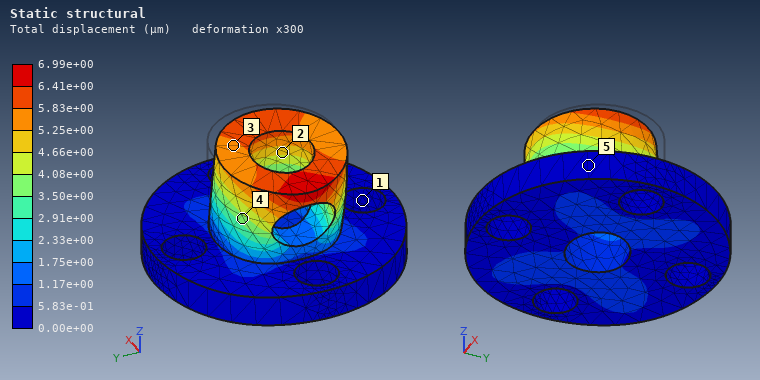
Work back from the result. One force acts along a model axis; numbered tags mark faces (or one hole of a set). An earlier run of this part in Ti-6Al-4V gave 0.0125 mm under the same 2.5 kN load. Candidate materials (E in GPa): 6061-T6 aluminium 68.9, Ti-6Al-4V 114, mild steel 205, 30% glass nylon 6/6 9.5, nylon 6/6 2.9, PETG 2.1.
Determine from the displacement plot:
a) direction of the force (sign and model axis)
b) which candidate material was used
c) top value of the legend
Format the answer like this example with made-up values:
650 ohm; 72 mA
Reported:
-X; mild steel; 6.99e+00 µm
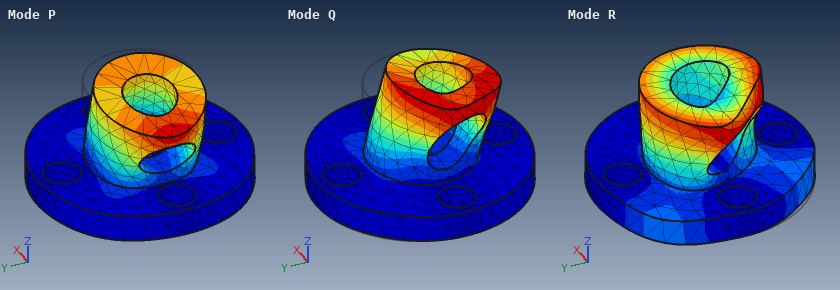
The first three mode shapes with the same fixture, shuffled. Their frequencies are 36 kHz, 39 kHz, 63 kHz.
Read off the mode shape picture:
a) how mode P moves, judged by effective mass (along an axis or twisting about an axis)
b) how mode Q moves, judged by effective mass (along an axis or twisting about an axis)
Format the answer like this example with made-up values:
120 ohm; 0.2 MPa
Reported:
along X; along Y
